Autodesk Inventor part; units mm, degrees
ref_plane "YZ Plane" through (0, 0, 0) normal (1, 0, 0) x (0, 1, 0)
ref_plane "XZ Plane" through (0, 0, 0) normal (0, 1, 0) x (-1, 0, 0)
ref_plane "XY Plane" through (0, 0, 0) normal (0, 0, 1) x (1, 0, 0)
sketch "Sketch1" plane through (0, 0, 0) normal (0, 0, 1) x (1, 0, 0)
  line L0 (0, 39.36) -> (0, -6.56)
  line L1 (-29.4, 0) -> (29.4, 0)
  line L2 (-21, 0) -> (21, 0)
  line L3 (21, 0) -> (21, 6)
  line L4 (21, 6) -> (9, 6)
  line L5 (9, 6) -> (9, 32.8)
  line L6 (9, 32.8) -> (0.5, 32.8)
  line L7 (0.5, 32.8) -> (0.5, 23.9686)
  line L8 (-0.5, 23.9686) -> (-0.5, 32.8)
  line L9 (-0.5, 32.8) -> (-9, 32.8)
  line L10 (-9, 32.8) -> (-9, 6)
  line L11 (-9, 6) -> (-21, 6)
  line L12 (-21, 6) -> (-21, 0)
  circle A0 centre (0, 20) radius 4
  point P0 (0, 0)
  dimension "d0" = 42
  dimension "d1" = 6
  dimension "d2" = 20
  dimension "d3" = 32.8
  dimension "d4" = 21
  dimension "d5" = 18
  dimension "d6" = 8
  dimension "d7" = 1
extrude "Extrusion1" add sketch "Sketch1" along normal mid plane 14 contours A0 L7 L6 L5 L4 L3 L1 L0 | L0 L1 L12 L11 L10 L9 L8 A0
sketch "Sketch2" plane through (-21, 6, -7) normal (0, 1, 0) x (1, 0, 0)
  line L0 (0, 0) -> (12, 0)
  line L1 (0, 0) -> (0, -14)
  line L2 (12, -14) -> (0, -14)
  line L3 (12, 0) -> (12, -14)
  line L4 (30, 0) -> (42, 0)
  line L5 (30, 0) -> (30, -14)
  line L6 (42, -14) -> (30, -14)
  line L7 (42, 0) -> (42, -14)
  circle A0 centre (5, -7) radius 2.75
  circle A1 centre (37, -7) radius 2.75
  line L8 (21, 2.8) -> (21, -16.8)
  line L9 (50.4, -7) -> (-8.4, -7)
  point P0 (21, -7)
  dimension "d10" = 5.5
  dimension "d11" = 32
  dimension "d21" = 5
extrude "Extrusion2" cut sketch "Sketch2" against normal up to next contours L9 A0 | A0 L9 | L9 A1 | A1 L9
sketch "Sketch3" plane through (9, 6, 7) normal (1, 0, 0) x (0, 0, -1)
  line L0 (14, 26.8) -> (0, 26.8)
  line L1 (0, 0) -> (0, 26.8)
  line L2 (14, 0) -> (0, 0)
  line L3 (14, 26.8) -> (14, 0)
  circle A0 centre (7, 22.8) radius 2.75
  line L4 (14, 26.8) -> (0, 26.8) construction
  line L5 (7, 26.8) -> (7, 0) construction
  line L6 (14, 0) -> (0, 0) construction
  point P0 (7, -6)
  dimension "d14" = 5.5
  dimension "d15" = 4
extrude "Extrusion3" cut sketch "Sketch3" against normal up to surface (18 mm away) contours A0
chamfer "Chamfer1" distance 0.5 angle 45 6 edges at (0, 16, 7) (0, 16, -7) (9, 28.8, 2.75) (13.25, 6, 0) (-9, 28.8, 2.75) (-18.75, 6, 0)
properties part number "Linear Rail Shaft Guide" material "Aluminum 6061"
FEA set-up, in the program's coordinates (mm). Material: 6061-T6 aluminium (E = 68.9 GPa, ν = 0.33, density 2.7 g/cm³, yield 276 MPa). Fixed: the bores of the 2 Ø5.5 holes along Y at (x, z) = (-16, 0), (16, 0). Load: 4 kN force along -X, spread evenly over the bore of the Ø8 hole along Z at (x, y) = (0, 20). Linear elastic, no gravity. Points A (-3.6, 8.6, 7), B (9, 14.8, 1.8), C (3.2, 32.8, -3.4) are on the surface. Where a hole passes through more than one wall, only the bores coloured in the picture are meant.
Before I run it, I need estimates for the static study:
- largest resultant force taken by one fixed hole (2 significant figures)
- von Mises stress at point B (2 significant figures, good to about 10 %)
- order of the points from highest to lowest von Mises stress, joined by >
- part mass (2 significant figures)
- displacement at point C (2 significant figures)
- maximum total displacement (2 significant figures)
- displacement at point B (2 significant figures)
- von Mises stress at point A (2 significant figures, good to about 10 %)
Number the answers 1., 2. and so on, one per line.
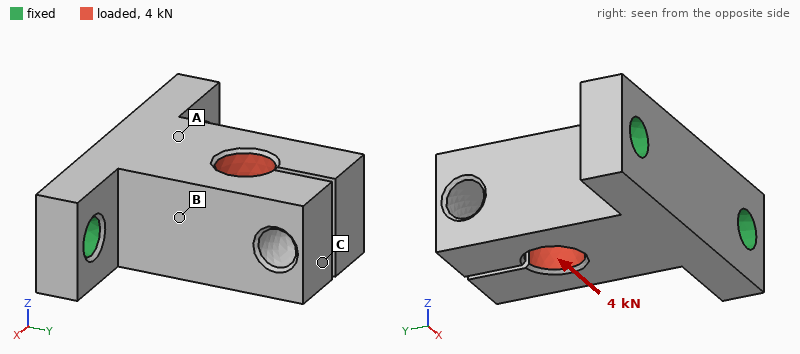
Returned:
1. 3.4 kN
2. 61 MPa
3. B > A > C
4. 24 g
5. 0.12 mm
6. 0.12 mm
7. 0.038 mm
8. 32 MPa
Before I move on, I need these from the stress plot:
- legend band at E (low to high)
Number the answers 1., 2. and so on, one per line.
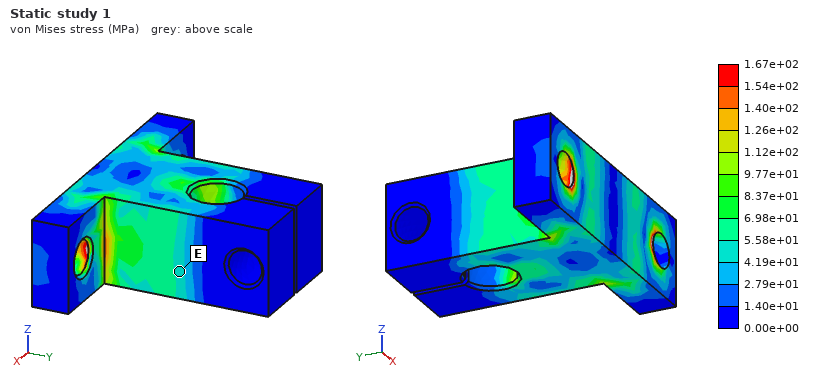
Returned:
1. 4.19e+01 to 5.58e+01 MPa
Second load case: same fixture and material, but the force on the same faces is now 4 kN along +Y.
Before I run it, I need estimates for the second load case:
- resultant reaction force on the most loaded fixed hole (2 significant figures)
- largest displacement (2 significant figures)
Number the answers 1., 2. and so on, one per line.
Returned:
1. 2.2 kN
2. 53 µm
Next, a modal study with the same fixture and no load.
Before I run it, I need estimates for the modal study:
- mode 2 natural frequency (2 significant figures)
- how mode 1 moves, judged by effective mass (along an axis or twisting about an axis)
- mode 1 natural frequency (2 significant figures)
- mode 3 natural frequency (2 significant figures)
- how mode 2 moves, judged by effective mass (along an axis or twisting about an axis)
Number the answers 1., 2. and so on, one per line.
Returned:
1. 8600 Hz
2. along Z
3. 5200 Hz
4. 11 kHz
5. along X
